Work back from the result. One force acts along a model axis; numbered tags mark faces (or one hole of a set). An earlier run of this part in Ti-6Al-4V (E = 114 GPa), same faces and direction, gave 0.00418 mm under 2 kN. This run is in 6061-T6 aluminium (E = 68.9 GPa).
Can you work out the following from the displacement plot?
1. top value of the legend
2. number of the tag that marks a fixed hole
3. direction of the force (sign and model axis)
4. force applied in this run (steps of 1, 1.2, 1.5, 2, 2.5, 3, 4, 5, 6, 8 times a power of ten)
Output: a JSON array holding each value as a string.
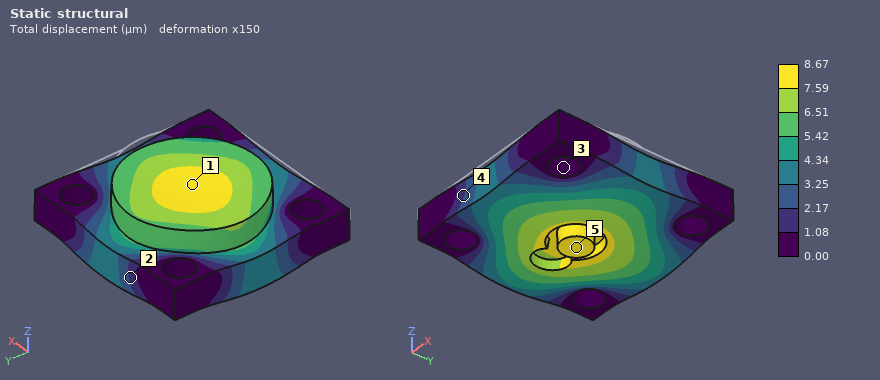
["8.67 µm", "3", "-Z", "2.5 kN"]
